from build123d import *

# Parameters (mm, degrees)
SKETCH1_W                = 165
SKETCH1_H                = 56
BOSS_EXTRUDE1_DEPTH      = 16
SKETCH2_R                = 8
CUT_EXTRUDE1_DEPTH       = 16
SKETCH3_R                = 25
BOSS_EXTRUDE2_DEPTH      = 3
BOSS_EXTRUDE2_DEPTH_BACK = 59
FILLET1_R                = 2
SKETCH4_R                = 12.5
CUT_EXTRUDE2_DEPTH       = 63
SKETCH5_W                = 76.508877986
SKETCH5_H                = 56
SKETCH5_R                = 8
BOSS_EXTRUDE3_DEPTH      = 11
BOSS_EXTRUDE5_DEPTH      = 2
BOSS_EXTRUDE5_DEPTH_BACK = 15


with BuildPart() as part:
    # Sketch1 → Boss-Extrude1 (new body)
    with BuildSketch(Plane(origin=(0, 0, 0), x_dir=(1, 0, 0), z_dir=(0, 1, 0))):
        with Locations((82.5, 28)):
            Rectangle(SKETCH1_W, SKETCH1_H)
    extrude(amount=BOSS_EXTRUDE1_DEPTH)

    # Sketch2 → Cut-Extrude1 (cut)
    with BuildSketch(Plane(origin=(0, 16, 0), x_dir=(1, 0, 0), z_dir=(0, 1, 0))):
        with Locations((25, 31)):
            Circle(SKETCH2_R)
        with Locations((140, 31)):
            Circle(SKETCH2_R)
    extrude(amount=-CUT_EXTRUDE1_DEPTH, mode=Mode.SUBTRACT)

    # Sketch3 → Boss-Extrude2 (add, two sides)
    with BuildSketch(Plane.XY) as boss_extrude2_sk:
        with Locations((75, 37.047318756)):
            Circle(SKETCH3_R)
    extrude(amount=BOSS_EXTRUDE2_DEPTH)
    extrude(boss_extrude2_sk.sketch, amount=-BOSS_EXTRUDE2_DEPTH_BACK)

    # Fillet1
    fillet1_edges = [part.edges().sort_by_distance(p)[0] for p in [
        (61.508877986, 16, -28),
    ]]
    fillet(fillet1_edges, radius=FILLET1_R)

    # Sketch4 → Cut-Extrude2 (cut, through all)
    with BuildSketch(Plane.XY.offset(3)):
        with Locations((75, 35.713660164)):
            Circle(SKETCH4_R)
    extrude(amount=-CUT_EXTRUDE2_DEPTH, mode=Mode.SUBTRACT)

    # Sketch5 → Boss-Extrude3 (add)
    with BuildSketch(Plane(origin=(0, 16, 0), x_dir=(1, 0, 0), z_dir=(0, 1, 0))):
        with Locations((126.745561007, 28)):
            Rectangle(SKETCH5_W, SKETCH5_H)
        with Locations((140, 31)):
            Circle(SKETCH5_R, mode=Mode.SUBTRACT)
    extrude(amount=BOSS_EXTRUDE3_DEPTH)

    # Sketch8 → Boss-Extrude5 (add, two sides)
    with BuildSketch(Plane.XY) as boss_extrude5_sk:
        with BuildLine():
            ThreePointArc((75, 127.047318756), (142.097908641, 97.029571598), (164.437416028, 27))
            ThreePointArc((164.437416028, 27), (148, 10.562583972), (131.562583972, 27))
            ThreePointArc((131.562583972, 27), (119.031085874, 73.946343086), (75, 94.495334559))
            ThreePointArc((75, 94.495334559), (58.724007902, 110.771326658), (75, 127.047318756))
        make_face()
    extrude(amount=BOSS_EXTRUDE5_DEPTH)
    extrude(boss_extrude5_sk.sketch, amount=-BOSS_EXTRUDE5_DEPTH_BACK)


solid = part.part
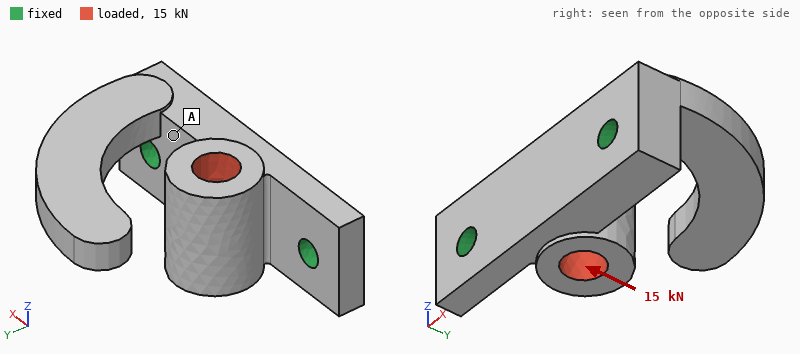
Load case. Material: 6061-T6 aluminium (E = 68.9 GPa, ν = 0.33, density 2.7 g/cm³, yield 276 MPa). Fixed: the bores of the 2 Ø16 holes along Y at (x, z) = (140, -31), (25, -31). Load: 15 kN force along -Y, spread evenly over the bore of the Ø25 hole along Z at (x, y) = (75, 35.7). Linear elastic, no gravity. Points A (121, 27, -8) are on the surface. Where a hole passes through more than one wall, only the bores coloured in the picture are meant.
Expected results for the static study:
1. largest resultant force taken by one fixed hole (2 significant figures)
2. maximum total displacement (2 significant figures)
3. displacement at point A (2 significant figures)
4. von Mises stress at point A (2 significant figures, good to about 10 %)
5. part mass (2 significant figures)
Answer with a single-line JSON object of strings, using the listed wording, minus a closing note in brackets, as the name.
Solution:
{"largest resultant force taken by one fixed hole": "7.9 kN", "maximum total displacement": "50 µm", "displacement at point A": "13 µm", "von Mises stress at point A": "11 MPa", "part mass": "940 g"}
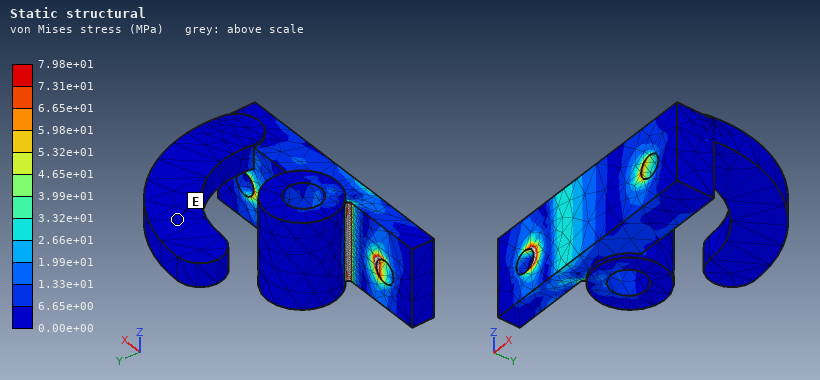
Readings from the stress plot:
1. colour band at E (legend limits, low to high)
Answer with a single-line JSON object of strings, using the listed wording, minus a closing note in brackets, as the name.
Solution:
{"colour band at E": "0.00e+00 to 6.65e+00 MPa"}
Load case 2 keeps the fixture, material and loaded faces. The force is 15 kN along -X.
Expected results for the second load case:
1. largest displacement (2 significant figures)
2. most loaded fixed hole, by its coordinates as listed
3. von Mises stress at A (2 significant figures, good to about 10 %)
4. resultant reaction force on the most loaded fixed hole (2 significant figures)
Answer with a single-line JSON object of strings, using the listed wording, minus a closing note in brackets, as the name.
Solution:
{"largest displacement": "46 µm", "most loaded fixed hole, by its coordinates as listed": "(140, -31)", "von Mises stress at A": "10 MPa", "resultant reaction force on the most loaded fixed hole": "11 kN"}
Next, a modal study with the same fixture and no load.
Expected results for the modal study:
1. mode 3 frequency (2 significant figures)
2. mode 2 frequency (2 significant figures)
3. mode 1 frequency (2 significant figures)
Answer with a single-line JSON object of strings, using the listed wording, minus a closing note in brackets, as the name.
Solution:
{"mode 3 frequency": "2500 Hz", "mode 2 frequency": "1100 Hz", "mode 1 frequency": "690 Hz"}
